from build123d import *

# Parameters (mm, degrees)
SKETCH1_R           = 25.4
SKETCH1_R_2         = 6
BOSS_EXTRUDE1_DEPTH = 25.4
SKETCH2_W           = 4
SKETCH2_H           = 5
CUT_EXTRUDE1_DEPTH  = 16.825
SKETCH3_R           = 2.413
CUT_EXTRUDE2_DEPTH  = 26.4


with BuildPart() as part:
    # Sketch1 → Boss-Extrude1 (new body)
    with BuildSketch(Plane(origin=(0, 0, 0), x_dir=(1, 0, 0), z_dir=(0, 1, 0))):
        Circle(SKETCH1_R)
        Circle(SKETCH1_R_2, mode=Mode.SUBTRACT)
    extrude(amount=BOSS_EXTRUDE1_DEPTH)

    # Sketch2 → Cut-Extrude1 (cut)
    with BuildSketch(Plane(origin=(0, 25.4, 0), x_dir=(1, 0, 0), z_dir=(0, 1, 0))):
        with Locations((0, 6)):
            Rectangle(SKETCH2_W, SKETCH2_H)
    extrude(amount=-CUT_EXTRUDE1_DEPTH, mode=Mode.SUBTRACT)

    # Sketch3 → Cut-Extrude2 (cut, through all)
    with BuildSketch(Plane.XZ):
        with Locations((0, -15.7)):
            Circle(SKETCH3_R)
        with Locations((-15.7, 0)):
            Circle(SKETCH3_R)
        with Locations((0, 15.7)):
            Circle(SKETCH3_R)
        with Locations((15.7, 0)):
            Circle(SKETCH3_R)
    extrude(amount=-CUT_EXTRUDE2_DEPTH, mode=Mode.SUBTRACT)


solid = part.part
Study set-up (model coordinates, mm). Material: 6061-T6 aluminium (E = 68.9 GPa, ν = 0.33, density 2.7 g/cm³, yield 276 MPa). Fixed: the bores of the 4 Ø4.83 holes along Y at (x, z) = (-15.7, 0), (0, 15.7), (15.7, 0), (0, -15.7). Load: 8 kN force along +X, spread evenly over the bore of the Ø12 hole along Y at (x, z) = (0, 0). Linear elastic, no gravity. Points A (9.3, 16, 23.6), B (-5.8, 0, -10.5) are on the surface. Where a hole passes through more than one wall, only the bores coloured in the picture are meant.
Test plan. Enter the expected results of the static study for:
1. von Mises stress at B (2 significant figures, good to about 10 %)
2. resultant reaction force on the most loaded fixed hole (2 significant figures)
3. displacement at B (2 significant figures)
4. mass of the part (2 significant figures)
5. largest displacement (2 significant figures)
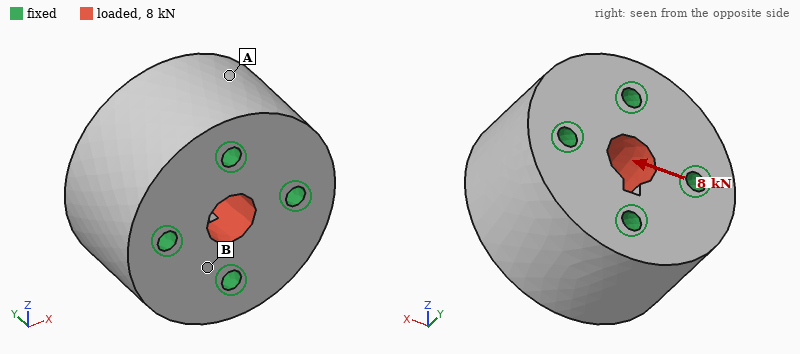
3.6 MPa
2.7 kN
0.65 µm
130 g
1.7 µm
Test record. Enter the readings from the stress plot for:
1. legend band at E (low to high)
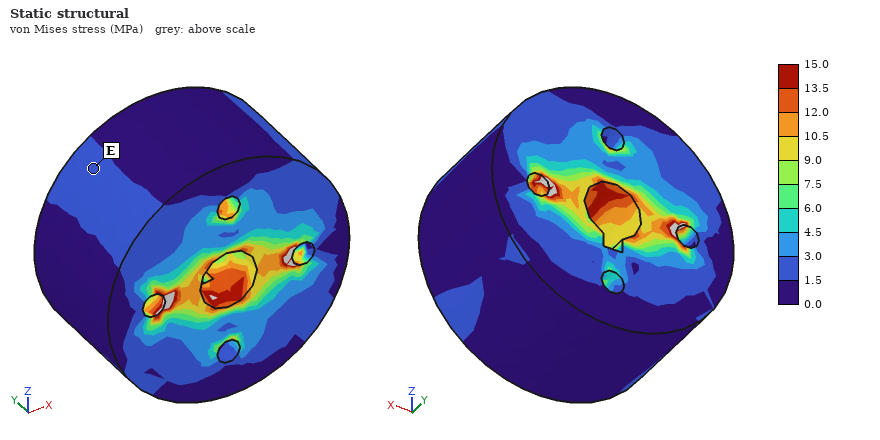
1.5 to 3.0 MPa
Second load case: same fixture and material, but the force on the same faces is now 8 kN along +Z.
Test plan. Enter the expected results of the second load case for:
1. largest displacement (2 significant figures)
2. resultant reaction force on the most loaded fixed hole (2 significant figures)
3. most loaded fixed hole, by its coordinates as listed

1.6 µm
2.8 kN
(0, 15.7)
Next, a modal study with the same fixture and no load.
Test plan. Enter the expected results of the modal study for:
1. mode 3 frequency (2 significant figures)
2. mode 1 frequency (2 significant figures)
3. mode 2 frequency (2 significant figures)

46 kHz
45 kHz
46 kHz
